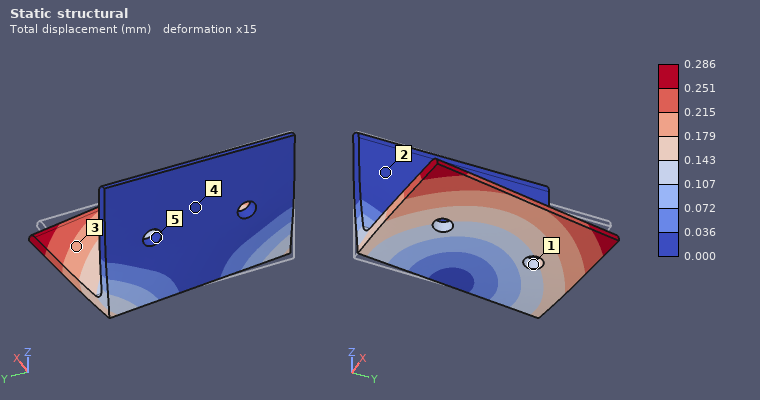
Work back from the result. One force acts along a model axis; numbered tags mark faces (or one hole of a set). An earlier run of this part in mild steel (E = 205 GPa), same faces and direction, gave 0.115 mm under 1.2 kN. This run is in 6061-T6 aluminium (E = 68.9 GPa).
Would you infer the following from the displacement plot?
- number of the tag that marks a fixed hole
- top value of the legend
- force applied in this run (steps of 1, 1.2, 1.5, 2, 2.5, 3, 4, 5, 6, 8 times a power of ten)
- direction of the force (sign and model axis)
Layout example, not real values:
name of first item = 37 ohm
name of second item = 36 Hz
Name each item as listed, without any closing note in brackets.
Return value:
number of the tag that marks a fixed hole = 5
top value of the legend = 0.286 mm
force applied in this run = 1 kN
direction of the force = +Y
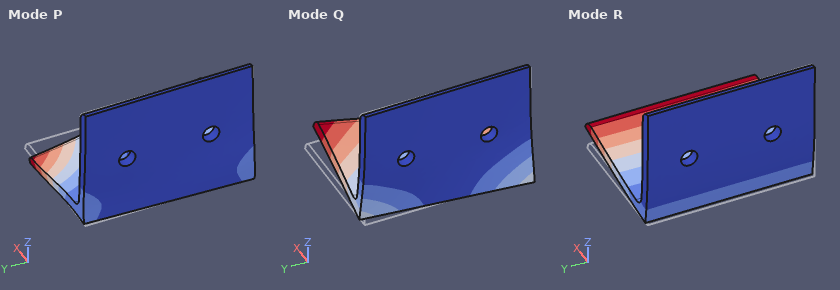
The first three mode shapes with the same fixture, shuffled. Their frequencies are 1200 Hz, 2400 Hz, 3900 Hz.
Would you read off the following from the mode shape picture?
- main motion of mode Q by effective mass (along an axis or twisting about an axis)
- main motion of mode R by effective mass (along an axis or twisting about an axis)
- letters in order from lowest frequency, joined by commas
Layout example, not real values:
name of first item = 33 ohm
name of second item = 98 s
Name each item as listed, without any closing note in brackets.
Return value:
main motion of mode Q by effective mass = along Y
main motion of mode R by effective mass = along Z
letters in order from lowest frequency, joined by commas = R, Q, P
